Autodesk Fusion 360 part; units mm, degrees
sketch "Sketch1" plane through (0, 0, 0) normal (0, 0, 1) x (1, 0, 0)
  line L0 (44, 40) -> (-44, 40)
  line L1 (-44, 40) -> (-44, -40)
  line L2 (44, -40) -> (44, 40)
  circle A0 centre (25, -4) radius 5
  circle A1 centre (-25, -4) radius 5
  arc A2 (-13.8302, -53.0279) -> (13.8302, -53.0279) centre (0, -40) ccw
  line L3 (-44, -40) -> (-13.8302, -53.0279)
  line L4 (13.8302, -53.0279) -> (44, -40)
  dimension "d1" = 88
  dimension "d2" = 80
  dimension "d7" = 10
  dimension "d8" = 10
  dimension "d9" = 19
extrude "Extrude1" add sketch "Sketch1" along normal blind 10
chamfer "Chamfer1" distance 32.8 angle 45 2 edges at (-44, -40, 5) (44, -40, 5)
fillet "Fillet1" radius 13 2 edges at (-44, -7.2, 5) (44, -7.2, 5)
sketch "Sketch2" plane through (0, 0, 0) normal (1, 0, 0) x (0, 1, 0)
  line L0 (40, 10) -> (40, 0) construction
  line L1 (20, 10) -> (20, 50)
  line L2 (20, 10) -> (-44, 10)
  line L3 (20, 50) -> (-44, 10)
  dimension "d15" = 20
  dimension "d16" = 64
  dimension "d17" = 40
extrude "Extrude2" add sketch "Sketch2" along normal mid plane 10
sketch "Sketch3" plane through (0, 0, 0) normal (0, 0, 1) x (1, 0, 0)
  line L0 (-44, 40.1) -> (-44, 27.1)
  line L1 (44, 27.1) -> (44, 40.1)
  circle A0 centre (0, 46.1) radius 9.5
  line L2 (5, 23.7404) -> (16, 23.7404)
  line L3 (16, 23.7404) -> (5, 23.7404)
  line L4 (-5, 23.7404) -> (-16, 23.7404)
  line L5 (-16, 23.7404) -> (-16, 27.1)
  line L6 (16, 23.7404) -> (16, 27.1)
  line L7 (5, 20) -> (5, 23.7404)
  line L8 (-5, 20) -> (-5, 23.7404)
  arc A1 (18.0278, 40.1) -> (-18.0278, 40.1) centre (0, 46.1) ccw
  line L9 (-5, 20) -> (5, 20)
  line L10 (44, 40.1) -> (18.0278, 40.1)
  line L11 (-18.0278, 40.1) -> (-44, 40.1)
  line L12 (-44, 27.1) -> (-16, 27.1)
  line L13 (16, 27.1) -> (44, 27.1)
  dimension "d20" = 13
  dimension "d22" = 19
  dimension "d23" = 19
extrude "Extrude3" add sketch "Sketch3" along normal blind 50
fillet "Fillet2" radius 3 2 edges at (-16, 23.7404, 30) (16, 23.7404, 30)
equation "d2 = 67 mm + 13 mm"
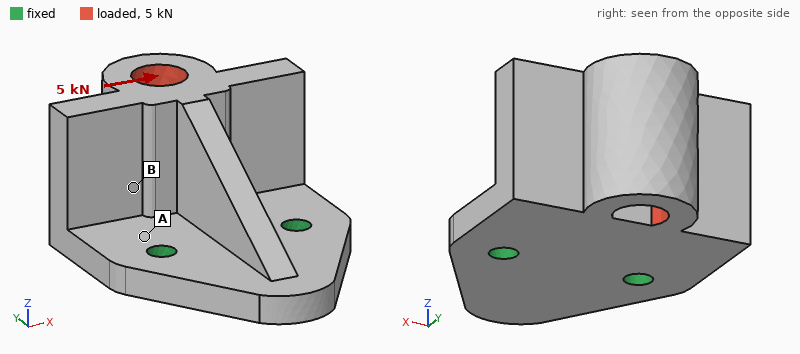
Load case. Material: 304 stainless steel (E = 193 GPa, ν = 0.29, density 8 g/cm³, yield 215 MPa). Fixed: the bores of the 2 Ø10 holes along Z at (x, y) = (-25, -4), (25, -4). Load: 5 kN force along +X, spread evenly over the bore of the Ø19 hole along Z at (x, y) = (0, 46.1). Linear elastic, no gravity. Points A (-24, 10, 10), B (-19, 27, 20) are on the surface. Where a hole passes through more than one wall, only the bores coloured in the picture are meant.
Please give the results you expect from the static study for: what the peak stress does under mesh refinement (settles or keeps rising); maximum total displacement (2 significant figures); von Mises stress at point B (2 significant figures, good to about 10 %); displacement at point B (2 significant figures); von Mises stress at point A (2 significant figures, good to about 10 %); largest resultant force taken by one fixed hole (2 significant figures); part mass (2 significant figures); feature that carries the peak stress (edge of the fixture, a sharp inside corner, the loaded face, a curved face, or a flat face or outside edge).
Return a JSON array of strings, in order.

["keeps rising", "27 µm", "7.7 MPa", "12 µm", "27 MPa", "5.5 kN", "1.3 kg", "edge of the fixture"]
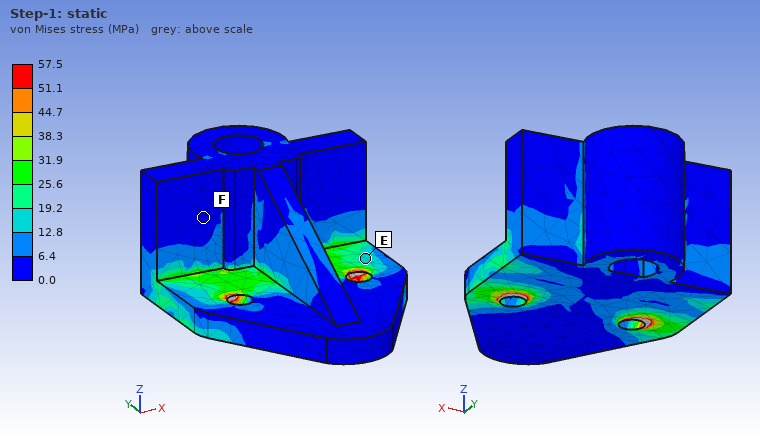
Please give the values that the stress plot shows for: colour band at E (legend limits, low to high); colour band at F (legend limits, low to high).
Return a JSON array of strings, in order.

["12.8 to 19.2 MPa", "0.0 to 6.4 MPa"]
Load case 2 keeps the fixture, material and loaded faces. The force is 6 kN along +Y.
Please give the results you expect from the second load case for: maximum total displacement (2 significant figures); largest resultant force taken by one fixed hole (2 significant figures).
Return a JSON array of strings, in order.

["64 µm", "3.0 kN"]
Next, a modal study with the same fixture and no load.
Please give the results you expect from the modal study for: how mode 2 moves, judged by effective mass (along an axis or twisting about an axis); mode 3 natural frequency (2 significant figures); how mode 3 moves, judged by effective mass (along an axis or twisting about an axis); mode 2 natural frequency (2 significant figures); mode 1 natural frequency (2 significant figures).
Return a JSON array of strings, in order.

["along X", "5300 Hz", "along Z", "2700 Hz", "1500 Hz"]
